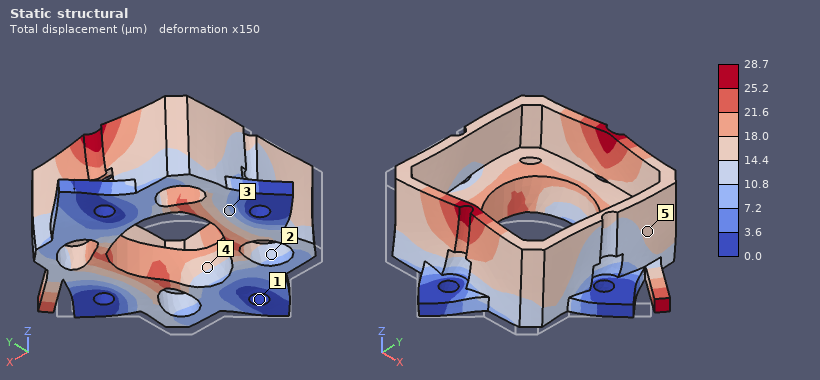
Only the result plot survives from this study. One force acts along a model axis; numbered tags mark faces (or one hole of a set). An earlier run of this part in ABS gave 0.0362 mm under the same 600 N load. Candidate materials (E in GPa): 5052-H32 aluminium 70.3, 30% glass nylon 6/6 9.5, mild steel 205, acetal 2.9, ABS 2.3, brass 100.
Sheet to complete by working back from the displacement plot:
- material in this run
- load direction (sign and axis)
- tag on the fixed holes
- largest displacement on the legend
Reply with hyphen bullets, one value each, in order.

- acetal
- +Y
- 1
- 28.7 µm
